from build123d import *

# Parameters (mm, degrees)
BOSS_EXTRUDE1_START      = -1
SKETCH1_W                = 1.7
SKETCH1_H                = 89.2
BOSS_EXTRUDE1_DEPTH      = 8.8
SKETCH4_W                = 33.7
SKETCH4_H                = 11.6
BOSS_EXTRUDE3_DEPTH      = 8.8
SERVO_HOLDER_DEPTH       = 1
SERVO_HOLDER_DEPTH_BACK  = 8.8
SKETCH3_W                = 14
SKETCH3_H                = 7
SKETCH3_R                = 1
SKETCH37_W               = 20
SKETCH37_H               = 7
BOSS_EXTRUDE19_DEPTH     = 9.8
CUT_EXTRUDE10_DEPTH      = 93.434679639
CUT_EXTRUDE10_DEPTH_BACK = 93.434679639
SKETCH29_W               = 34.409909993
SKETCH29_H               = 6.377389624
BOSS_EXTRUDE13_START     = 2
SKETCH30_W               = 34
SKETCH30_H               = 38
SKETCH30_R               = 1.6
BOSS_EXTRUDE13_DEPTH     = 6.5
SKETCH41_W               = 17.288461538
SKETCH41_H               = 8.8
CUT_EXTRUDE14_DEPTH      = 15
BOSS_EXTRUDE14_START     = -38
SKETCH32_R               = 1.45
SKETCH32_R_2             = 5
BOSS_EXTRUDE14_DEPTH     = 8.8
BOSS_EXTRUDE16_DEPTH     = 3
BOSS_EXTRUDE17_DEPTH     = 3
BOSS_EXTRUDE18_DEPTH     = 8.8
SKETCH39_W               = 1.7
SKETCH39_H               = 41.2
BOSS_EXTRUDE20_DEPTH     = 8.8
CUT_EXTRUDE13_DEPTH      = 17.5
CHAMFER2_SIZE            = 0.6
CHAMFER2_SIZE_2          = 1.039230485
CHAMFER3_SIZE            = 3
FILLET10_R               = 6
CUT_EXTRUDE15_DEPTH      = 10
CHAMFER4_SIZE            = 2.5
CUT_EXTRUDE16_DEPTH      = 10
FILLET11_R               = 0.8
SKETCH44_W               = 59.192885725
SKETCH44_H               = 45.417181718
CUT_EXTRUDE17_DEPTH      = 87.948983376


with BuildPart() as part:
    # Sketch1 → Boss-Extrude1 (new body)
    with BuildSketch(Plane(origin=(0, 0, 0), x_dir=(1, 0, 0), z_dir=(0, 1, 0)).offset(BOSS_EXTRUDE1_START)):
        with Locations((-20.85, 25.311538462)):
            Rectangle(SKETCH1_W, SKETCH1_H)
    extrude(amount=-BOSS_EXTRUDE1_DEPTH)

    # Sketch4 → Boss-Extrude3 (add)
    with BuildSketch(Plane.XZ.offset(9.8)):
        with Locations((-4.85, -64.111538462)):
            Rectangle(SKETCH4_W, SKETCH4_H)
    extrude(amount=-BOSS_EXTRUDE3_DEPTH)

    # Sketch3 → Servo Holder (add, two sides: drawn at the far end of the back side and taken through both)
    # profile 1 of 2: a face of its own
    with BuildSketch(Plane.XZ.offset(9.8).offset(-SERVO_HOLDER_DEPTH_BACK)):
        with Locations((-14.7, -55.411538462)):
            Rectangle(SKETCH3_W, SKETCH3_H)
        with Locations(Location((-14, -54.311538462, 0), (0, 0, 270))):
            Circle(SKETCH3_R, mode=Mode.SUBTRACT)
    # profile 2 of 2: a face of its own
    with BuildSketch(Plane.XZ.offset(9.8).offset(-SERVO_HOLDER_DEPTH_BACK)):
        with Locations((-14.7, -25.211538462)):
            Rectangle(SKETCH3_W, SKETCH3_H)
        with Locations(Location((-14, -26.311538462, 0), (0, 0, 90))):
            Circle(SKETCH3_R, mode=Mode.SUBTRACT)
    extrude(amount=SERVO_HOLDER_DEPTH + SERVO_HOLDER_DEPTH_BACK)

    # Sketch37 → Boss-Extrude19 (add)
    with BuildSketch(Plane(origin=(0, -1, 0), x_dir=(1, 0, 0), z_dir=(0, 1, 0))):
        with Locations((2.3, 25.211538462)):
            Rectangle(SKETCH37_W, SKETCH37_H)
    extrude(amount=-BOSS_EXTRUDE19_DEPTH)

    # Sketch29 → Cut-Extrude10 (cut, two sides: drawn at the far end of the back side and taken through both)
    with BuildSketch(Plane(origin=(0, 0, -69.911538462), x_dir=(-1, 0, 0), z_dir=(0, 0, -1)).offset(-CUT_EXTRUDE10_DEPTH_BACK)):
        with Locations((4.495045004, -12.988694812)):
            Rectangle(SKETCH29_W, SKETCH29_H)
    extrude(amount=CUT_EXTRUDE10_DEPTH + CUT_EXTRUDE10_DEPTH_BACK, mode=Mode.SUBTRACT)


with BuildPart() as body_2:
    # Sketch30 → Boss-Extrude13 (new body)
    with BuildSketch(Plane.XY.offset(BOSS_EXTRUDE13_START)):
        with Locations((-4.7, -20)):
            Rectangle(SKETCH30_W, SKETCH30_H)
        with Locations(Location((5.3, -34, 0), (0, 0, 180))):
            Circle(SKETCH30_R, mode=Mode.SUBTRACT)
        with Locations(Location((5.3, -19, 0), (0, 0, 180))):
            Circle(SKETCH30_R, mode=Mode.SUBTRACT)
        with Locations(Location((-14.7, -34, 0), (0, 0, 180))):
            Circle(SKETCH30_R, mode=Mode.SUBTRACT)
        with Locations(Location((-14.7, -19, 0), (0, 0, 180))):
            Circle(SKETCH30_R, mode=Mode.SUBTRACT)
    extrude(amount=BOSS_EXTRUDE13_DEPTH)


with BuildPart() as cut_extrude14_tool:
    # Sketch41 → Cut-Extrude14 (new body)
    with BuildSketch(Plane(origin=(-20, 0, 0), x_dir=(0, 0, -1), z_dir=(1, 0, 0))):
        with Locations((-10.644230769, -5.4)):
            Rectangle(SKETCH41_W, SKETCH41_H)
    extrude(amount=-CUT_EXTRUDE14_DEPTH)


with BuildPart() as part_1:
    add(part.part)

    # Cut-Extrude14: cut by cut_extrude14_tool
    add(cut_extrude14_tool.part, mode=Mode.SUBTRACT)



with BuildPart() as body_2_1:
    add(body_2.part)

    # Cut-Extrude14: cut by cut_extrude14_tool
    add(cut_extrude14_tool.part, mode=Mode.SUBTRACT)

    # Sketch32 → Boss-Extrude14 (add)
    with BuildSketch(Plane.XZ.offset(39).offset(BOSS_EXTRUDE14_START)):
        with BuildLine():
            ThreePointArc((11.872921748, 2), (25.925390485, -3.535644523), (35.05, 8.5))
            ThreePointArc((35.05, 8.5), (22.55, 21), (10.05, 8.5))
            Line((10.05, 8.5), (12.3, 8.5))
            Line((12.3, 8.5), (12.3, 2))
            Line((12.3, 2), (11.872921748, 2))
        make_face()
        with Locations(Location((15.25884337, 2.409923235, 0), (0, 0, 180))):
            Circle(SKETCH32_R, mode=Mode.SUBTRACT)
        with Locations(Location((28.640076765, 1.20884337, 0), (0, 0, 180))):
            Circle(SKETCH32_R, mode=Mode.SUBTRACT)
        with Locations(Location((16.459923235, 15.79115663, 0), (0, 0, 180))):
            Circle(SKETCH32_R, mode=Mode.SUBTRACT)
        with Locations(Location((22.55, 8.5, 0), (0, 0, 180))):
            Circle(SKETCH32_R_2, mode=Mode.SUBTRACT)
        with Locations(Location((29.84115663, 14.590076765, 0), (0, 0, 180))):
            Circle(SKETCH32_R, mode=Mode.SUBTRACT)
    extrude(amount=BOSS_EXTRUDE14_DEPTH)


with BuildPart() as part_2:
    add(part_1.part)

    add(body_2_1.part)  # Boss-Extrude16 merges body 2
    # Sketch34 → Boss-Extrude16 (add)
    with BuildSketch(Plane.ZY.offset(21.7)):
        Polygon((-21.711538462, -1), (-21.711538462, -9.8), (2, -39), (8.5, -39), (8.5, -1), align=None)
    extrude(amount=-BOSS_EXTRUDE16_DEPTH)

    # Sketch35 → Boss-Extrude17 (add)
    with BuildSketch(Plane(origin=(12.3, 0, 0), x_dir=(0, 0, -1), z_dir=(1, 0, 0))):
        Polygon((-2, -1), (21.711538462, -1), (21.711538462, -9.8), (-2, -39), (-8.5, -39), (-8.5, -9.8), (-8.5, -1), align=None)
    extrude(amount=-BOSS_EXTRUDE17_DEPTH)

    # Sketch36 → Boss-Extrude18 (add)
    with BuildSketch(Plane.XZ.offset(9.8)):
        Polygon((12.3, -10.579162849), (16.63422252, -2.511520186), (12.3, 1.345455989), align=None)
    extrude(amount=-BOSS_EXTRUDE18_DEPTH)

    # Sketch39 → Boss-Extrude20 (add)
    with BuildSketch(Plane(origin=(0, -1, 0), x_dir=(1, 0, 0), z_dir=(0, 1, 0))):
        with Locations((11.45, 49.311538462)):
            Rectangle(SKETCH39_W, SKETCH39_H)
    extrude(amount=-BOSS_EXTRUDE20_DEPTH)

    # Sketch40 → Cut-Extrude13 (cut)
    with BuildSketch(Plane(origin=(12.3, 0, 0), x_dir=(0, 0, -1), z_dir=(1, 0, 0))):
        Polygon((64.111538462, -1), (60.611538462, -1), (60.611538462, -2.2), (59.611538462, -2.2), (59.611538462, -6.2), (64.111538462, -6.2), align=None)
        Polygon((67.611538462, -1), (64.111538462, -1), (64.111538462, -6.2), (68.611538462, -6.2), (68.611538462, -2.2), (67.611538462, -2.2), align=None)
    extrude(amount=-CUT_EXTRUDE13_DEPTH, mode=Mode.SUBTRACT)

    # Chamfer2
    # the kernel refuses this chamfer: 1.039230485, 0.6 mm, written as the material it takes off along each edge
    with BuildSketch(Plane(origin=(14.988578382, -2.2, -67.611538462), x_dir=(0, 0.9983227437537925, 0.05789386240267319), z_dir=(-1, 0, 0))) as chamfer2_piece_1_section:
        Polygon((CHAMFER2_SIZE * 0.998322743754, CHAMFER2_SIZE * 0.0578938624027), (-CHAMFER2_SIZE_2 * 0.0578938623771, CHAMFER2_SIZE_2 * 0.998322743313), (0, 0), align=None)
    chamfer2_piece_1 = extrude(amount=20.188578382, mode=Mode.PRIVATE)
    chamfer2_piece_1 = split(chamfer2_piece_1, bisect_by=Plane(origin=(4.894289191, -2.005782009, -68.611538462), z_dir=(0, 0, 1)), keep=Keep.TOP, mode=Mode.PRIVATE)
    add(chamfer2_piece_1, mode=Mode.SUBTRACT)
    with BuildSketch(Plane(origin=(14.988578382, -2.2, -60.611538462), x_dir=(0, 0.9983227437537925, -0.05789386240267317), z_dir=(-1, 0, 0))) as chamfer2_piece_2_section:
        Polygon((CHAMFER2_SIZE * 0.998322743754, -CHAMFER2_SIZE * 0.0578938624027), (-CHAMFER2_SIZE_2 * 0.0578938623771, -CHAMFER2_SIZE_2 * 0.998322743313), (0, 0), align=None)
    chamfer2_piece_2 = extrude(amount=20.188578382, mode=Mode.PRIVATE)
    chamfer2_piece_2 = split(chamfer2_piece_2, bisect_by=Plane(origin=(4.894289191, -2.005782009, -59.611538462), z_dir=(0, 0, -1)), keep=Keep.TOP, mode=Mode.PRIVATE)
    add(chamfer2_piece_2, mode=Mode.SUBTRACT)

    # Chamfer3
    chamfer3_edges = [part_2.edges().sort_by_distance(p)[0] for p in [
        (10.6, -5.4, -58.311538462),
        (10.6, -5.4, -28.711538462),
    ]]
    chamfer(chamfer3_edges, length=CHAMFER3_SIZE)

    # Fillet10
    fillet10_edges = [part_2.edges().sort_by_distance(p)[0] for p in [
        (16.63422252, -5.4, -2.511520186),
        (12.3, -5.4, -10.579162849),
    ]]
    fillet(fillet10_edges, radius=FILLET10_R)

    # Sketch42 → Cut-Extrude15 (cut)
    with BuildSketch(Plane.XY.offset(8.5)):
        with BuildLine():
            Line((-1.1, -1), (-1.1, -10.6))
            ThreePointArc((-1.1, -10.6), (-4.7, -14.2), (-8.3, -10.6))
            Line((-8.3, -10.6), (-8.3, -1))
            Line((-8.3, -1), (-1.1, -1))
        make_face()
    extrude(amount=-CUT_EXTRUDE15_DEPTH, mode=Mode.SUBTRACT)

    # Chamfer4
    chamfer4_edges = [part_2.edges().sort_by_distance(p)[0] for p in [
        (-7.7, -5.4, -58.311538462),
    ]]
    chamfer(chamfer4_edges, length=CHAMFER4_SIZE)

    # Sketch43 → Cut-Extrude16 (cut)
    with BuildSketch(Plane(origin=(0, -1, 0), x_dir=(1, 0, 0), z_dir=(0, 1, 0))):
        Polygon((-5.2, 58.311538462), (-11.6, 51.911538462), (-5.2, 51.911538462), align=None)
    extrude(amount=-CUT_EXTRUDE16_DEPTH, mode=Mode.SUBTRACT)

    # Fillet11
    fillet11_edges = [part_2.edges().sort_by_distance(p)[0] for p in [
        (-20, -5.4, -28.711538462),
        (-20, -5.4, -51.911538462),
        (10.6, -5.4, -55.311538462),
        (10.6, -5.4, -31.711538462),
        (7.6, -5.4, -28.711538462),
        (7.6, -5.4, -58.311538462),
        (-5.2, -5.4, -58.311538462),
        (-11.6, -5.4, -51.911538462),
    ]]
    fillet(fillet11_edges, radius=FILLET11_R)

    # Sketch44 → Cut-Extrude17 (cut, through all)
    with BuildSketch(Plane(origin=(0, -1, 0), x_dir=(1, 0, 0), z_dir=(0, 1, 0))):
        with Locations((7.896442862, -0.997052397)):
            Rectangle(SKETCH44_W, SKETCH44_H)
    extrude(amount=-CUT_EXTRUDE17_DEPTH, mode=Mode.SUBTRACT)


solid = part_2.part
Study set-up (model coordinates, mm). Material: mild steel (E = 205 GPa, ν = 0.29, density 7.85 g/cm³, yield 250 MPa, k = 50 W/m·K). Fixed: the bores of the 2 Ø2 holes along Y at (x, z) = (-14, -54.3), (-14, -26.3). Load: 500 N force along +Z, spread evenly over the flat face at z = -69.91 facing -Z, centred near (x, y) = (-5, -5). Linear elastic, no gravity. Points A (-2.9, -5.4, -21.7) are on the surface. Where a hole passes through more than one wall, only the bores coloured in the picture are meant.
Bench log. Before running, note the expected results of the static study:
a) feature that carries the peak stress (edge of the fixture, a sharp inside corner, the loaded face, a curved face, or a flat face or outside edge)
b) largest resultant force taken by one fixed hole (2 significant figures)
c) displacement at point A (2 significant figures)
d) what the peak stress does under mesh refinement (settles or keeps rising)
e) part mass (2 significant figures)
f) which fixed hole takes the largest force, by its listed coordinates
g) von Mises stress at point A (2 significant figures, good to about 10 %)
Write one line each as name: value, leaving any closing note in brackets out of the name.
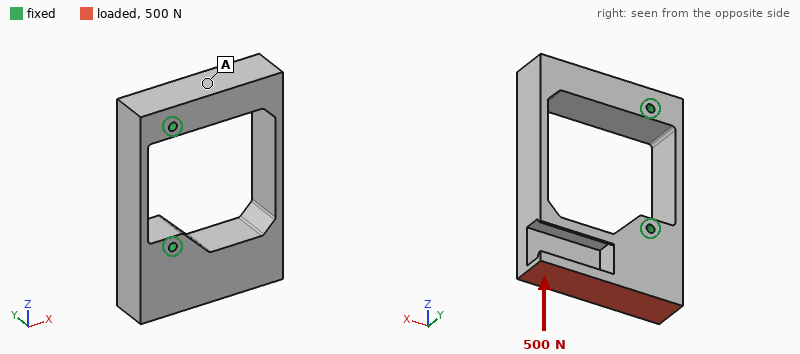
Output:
feature that carries the peak stress: edge of the fixture
largest resultant force taken by one fixed hole: 500 N
displacement at point A: 3.8 µm
what the peak stress does under mesh refinement: keeps rising
part mass: 50 g
which fixed hole takes the largest force, by its listed coordinates: (-14, -54.3)
von Mises stress at point A: 10 MPa
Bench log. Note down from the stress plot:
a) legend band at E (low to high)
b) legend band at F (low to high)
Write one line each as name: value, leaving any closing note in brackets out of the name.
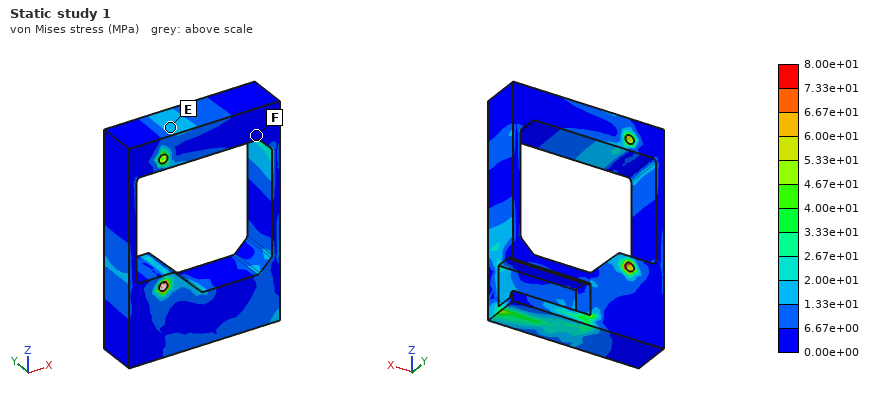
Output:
legend band at E: 1.33e+01 to 2.00e+01 MPa
legend band at F: 0.00e+00 to 6.67e+00 MPa
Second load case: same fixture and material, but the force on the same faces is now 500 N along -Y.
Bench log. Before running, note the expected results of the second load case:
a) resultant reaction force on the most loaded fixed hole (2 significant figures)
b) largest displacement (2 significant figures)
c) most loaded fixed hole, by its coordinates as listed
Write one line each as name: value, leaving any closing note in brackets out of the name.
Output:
resultant reaction force on the most loaded fixed hole: 530 N
largest displacement: 26 µm
most loaded fixed hole, by its coordinates as listed: (-14, -54.3)
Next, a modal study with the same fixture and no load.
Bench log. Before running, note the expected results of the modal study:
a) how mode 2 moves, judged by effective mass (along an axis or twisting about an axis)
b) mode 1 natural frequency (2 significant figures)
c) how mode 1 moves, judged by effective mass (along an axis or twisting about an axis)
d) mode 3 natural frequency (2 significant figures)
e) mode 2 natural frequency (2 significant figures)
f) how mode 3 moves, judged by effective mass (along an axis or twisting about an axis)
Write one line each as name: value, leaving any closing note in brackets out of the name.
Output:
how mode 2 moves, judged by effective mass: along Y
mode 1 natural frequency: 5300 Hz
how mode 1 moves, judged by effective mass: along Z
mode 3 natural frequency: 8800 Hz
mode 2 natural frequency: 7100 Hz
how mode 3 moves, judged by effective mass: twisting about X
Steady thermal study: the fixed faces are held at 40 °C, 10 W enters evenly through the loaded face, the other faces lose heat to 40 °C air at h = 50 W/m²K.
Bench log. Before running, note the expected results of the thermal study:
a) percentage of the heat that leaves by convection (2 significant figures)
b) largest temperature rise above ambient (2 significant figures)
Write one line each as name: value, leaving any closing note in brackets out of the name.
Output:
percentage of the heat that leaves by convection: 19 %
largest temperature rise above ambient: 39 K
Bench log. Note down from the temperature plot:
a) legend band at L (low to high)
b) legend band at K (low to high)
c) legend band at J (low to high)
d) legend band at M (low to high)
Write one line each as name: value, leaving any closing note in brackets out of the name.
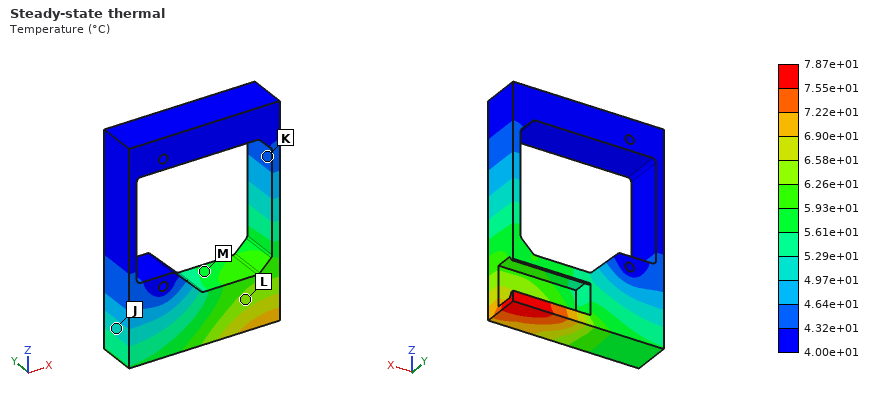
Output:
legend band at L: 6.26e+01 to 6.58e+01 °C
legend band at K: 4.32e+01 to 4.64e+01 °C
legend band at J: 4.97e+01 to 5.29e+01 °C
legend band at M: 5.61e+01 to 5.93e+01 °C
